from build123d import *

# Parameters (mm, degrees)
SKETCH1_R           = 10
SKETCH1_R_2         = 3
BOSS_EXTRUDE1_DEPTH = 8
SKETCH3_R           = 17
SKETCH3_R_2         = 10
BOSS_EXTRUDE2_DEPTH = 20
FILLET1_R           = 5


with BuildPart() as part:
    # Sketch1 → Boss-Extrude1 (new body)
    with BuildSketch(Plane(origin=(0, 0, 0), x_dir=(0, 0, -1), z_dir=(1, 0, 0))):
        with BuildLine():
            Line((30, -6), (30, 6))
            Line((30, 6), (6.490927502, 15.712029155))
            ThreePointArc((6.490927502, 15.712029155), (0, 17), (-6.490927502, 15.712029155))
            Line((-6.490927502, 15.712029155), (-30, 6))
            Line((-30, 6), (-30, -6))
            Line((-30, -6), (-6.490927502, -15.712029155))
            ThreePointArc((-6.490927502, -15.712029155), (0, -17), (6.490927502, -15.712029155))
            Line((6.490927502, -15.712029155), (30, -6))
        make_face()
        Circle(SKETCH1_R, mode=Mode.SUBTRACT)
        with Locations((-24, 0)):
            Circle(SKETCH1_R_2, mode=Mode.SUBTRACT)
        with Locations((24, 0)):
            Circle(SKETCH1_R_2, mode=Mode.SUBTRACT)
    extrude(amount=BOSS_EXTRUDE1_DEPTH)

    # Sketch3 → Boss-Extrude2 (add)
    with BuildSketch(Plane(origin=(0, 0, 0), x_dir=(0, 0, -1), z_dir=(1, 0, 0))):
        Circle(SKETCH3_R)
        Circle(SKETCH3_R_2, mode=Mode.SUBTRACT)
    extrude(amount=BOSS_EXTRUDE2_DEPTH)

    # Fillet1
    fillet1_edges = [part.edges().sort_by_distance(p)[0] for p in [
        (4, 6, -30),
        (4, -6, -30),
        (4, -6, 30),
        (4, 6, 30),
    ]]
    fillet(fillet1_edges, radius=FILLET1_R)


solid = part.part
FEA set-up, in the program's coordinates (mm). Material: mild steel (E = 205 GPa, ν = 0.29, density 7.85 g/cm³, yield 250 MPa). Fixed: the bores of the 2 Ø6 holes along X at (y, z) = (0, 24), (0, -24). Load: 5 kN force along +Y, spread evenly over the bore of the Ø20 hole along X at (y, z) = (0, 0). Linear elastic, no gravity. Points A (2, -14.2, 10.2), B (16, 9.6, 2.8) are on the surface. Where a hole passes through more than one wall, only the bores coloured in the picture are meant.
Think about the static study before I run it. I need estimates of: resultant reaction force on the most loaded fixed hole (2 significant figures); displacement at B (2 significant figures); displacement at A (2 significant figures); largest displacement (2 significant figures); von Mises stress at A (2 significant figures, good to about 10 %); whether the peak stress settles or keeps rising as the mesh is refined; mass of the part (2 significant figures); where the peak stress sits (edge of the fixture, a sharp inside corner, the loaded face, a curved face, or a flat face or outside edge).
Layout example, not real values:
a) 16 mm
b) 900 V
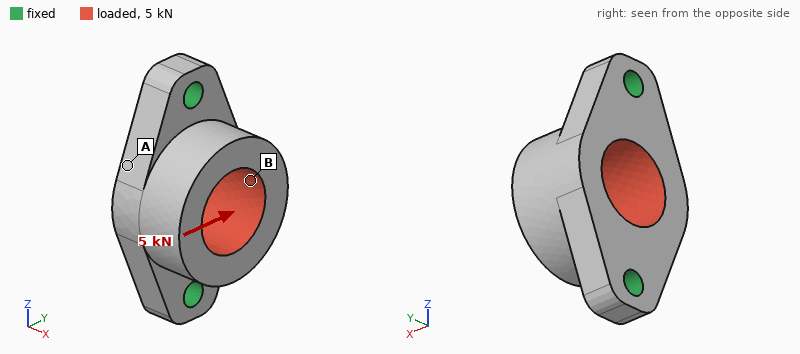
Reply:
a) 2.5 kN
b) 13 µm
c) 8.7 µm
d) 18 µm
e) 29 MPa
f) keeps rising
g) 120 g
h) edge of the fixture
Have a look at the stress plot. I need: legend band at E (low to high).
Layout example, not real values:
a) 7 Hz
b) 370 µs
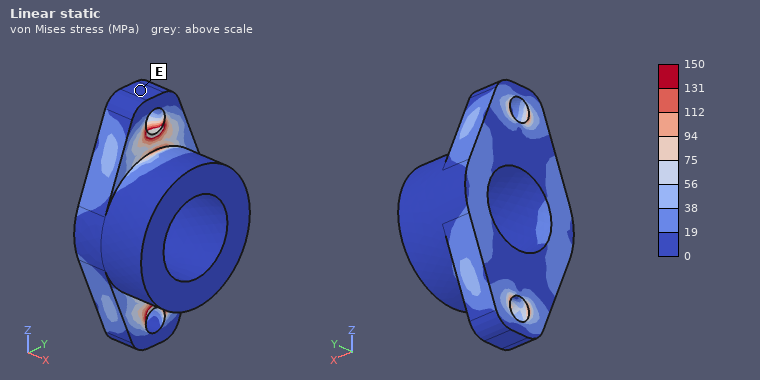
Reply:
a) 0 to 19 MPa
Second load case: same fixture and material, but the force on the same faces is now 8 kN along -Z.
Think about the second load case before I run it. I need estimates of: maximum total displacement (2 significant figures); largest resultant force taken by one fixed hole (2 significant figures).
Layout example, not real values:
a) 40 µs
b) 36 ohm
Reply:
a) 4.6 µm
b) 4.2 kN
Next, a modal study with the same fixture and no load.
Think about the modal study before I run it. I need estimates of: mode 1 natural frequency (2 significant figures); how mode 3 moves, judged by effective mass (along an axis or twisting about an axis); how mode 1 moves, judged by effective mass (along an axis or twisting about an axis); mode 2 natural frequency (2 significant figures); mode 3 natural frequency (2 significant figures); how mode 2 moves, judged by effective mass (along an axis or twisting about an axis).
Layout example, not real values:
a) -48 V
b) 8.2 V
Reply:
a) 8400 Hz
b) along Y
c) along Y
d) 14 kHz
e) 23 kHz
f) along X
